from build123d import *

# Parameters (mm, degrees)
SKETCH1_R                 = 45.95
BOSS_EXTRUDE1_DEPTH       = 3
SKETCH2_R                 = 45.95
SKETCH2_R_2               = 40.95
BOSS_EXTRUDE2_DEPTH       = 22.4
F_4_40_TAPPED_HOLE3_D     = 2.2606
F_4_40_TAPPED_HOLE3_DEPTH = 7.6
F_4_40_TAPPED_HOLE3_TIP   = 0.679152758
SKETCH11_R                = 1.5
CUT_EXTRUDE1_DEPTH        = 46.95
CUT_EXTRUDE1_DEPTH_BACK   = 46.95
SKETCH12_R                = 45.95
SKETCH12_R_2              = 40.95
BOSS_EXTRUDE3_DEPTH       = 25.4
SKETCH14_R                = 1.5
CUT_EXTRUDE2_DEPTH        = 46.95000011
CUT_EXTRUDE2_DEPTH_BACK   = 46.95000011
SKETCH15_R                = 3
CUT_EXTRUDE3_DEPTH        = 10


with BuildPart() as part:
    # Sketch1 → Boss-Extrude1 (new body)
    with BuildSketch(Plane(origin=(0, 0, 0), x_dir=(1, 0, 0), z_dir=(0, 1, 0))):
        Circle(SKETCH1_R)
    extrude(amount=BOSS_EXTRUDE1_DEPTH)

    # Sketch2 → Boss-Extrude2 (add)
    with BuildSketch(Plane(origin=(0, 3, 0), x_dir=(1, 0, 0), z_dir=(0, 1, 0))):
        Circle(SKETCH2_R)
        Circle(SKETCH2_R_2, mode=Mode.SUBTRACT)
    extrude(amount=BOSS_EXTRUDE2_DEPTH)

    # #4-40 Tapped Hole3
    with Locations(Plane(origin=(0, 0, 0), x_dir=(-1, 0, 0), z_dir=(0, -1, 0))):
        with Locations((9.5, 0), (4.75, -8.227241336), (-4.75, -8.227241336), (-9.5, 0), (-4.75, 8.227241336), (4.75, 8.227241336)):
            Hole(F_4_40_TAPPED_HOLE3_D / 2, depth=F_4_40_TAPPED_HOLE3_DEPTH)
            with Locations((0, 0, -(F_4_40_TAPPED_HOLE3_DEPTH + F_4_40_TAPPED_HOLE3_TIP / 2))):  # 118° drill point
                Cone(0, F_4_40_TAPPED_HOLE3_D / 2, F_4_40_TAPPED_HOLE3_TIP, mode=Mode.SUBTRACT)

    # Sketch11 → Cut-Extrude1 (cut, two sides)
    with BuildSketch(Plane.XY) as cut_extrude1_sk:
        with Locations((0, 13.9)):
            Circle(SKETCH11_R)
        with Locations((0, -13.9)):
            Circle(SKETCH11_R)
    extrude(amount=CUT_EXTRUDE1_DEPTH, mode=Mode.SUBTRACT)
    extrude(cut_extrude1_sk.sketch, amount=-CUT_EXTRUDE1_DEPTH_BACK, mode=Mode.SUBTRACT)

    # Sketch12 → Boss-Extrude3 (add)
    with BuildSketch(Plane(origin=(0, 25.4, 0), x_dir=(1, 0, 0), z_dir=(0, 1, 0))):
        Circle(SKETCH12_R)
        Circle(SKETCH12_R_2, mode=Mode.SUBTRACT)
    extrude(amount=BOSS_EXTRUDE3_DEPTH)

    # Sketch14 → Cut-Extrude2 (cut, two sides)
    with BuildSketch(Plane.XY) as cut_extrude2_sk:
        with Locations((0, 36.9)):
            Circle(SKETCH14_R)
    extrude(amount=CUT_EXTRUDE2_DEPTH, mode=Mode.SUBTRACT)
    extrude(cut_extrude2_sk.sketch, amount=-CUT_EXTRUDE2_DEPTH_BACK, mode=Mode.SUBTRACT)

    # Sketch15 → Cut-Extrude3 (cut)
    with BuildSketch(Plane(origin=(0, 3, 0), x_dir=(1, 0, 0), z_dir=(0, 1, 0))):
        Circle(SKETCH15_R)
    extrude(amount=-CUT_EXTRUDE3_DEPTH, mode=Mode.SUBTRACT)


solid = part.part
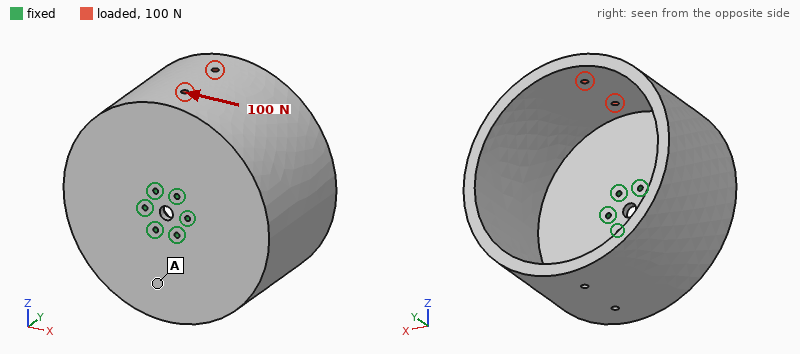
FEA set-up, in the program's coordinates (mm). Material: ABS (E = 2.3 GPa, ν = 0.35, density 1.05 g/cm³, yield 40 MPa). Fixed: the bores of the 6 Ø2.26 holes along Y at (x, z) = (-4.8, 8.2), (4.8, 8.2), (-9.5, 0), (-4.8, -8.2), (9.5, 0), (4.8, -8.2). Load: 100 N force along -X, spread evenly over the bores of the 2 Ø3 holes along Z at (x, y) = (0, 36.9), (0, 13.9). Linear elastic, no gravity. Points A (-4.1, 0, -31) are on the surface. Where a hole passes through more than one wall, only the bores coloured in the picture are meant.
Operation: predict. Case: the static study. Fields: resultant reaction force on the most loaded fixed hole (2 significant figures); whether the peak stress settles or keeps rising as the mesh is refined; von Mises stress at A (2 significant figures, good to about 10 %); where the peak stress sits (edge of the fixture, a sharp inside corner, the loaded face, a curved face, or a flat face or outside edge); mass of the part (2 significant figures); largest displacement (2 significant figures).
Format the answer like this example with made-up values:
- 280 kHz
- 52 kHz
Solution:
- 96 N
- keeps rising
- 1.9 MPa
- edge of the fixture
- 89 g
- 1.5 mm
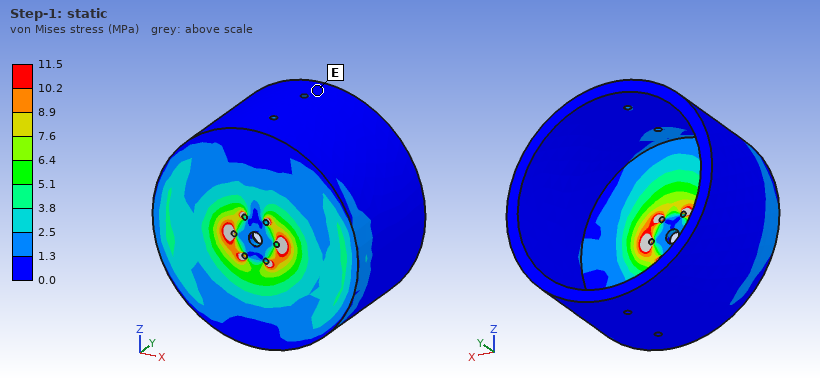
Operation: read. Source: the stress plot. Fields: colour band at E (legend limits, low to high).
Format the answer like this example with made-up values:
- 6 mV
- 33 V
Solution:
- 0.0 to 1.3 MPa
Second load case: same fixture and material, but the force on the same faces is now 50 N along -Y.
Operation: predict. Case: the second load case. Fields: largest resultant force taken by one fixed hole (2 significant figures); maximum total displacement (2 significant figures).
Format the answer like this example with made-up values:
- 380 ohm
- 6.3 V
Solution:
- 47 N
- 1.5 mm
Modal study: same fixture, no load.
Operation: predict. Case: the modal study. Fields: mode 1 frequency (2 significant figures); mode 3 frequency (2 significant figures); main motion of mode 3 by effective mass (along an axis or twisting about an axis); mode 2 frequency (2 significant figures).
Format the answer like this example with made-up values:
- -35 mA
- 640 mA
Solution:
- 150 Hz
- 310 Hz
- along Y
- 150 Hz
